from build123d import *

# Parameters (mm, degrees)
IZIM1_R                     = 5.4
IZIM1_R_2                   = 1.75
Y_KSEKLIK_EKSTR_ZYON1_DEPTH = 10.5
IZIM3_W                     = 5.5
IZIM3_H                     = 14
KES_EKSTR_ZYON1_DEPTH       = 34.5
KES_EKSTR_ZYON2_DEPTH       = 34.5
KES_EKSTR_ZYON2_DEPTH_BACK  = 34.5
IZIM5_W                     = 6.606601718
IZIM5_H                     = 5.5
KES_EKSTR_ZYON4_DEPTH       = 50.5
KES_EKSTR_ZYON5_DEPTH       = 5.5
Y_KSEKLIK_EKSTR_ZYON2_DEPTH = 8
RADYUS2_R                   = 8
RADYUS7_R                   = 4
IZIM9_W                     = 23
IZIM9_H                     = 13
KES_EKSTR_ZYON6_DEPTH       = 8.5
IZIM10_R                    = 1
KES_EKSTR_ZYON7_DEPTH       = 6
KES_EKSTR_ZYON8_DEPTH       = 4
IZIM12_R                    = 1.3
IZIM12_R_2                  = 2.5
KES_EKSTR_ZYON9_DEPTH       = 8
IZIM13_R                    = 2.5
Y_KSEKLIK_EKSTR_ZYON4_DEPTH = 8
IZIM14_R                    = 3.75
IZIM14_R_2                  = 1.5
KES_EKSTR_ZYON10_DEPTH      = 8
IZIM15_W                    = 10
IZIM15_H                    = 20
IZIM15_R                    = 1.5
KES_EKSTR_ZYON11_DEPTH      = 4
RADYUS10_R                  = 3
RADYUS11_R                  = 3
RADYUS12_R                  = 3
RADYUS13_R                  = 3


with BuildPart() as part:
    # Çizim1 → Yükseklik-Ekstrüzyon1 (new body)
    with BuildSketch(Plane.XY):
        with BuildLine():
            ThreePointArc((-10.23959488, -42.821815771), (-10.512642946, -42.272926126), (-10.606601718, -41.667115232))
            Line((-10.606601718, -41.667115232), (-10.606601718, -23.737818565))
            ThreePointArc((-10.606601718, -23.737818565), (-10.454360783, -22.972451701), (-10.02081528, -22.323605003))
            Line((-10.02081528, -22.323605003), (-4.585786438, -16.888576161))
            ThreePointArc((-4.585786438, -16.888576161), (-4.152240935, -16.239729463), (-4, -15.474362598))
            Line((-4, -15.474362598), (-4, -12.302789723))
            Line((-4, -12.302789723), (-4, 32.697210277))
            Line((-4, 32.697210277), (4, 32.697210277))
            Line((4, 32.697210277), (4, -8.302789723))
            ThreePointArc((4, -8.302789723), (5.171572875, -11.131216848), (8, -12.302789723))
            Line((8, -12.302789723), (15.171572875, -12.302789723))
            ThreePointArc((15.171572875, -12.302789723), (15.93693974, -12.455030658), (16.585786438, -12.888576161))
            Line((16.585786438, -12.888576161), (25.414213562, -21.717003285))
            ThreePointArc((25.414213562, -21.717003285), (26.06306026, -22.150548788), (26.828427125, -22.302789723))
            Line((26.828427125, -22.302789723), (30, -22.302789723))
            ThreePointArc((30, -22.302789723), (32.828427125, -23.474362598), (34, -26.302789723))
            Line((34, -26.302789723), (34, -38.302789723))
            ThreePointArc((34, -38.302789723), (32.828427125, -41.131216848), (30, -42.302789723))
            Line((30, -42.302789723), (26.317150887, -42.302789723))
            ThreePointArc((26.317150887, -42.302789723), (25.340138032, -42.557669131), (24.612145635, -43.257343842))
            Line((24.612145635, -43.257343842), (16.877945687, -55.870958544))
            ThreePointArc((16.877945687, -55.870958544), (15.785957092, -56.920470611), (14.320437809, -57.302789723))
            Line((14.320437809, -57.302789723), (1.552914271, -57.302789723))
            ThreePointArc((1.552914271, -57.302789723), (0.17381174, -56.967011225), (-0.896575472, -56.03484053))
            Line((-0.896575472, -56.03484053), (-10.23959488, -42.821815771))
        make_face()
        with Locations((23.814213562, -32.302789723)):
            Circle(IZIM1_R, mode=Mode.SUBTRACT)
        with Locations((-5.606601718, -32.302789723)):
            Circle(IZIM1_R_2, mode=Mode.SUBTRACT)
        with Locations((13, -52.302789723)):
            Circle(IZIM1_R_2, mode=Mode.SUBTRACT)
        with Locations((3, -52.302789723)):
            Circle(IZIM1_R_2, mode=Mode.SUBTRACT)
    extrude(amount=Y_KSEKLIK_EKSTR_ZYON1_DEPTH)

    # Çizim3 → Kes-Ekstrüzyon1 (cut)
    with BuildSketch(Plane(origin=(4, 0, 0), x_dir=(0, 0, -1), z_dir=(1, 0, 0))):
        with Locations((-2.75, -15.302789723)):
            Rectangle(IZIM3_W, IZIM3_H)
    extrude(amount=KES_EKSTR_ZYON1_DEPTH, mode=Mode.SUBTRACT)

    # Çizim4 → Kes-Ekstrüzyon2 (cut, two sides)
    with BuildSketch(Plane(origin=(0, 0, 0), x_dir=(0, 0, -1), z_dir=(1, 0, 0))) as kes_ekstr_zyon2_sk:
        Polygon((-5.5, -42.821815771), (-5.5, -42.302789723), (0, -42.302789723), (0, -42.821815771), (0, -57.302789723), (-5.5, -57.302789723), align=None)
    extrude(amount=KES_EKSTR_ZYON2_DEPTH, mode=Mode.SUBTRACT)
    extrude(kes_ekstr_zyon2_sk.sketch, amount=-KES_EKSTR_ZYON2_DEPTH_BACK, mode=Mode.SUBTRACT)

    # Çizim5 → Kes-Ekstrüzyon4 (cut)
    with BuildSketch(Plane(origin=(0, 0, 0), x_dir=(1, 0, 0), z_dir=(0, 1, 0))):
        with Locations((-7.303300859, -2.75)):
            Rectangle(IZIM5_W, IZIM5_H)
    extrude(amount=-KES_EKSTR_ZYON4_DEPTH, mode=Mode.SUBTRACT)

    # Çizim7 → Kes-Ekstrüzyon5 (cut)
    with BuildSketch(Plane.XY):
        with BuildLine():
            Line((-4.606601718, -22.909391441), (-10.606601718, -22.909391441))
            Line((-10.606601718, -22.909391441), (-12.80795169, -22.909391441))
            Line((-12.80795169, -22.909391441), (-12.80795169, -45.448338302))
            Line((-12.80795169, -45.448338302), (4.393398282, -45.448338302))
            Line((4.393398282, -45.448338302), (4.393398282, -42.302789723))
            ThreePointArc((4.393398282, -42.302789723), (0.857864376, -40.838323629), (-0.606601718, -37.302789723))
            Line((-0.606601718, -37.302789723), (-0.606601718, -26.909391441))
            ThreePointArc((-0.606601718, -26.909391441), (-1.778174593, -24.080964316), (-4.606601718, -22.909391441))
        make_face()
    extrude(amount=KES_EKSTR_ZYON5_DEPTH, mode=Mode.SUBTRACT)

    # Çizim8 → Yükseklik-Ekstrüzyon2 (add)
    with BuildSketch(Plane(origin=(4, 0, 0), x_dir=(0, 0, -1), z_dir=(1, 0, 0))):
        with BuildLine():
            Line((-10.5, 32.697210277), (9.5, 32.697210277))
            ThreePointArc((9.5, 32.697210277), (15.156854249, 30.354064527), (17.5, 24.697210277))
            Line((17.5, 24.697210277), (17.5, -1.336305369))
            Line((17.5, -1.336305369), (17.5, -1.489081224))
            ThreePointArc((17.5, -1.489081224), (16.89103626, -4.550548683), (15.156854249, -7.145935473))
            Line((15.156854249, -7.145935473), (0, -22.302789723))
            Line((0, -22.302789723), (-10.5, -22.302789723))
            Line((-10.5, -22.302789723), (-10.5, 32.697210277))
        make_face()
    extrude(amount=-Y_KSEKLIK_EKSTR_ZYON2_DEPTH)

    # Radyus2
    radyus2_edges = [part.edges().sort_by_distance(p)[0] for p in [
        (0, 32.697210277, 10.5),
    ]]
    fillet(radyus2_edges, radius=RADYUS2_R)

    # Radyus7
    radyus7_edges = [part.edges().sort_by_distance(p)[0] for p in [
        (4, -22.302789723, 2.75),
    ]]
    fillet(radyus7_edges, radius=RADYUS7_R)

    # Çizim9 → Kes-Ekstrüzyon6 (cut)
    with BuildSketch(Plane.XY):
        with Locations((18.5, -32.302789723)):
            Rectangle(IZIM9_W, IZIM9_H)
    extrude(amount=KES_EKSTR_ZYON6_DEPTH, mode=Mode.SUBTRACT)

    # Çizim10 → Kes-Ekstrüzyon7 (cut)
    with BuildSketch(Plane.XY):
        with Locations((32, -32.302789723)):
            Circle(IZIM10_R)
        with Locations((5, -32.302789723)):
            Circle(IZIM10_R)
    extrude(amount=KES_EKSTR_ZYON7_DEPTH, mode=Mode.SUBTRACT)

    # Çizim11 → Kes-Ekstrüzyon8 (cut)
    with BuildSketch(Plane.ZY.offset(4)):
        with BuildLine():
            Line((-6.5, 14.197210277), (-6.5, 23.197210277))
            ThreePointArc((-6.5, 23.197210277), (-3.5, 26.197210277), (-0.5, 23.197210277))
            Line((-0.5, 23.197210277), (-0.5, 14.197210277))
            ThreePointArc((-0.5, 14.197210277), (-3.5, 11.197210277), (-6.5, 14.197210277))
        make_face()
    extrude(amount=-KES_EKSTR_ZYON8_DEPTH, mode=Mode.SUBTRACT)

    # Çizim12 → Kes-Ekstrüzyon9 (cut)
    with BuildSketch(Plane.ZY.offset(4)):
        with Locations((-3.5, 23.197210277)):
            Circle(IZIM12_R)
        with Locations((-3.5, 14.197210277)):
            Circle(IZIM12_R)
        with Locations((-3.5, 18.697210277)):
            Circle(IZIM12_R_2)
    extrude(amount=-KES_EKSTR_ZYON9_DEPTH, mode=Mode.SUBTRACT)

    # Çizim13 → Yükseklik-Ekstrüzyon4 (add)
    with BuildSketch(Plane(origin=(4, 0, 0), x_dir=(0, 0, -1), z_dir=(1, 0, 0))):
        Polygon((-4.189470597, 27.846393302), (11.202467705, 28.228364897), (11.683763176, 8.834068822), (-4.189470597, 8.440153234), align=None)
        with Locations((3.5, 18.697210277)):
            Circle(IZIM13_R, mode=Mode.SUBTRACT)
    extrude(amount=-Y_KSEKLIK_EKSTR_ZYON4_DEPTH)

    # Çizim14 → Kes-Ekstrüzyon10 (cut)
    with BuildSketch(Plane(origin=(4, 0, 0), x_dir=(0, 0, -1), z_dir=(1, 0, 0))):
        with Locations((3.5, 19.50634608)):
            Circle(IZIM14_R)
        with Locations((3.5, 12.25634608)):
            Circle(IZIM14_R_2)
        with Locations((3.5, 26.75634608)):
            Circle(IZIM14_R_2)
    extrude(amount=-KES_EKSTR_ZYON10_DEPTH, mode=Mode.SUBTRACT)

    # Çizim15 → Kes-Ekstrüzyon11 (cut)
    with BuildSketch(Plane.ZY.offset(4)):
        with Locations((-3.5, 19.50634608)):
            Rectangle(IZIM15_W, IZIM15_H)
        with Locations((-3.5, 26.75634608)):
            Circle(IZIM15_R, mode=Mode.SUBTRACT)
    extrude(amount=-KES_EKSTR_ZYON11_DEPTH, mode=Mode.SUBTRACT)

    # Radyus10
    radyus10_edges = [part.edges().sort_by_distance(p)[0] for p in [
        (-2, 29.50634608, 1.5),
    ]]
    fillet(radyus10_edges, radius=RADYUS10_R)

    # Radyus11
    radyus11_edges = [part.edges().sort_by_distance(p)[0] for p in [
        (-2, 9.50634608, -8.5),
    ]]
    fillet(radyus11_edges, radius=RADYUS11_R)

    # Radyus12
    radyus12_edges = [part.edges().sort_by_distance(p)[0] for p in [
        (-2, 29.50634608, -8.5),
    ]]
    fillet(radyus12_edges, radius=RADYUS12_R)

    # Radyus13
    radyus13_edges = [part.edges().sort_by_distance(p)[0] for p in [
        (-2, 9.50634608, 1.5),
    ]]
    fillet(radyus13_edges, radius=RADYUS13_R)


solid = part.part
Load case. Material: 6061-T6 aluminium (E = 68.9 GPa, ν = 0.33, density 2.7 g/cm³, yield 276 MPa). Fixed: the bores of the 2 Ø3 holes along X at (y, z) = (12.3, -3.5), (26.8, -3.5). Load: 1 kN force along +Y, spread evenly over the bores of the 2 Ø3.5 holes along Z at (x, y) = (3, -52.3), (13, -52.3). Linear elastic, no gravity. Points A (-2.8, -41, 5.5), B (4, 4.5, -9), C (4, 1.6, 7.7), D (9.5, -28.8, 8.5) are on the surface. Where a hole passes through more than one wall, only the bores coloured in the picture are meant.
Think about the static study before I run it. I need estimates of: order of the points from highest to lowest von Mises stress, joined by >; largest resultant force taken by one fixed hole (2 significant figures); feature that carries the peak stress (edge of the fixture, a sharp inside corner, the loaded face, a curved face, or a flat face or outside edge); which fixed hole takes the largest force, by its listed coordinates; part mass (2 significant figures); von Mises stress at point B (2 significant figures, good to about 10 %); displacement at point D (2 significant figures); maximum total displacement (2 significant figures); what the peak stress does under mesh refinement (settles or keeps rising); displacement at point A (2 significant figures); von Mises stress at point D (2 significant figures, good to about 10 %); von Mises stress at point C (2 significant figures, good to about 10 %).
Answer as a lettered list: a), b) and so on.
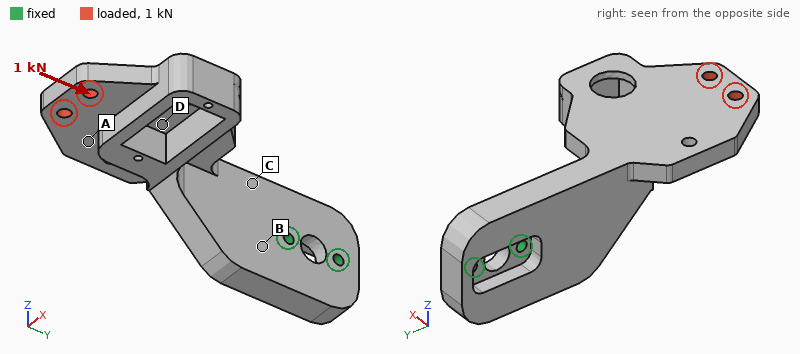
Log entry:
a) C > B > D > A
b) 1.1 kN
c) edge of the fixture
d) (12.3, -3.5)
e) 49 g
f) 26 MPa
g) 0.14 mm
h) 0.27 mm
i) keeps rising
j) 0.18 mm
k) 17 MPa
l) 44 MPa
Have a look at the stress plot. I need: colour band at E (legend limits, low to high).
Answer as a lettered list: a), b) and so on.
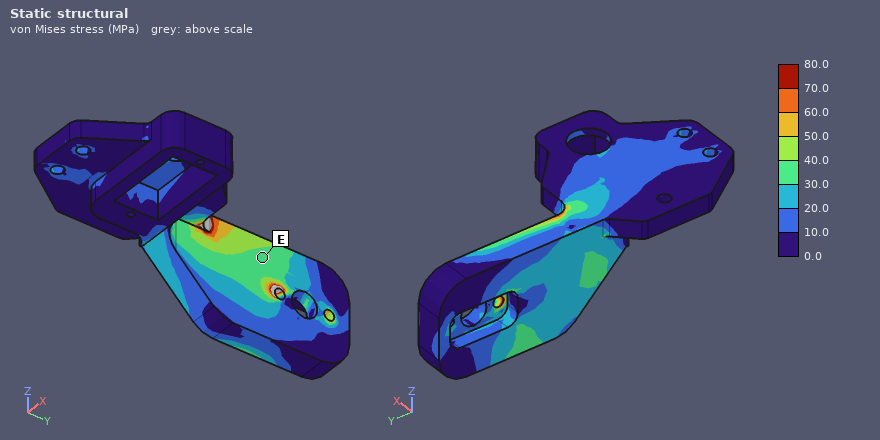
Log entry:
a) 30.0 to 40.0 MPa
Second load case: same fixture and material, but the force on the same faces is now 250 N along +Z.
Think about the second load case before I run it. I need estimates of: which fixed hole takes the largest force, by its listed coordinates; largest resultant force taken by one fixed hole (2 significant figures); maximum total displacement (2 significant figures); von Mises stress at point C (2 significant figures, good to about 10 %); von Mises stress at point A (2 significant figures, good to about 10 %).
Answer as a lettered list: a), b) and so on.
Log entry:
a) (12.3, -3.5)
b) 1.1 kN
c) 0.18 mm
d) 14 MPa
e) 13 MPa
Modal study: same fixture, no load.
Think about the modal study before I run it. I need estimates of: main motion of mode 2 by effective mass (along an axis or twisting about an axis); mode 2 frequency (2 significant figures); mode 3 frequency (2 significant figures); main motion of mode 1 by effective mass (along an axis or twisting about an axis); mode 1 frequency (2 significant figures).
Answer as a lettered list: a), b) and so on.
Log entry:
a) along Z
b) 1900 Hz
c) 3300 Hz
d) along X
e) 1100 Hz
